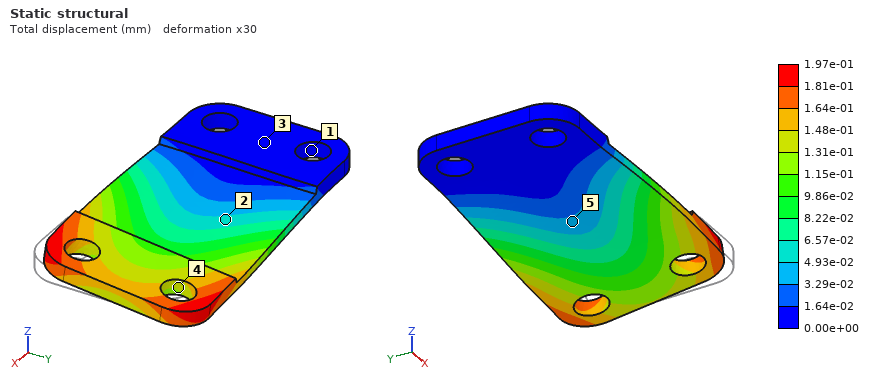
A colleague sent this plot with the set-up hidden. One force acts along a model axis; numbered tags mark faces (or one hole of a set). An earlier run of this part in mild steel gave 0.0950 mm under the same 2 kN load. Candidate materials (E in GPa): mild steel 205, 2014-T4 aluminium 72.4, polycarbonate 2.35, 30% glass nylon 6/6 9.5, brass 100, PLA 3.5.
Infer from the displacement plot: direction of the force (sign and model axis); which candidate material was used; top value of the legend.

+Y
brass
1.97e-01 mm
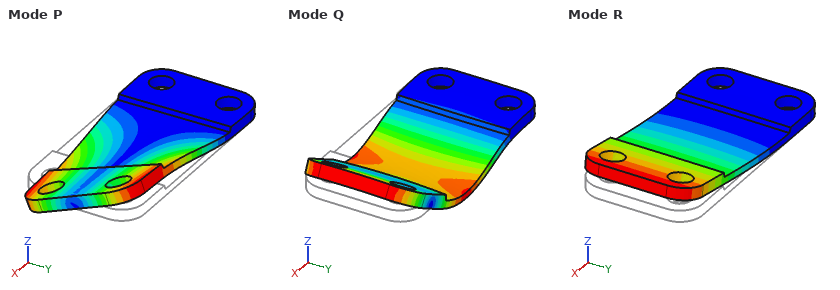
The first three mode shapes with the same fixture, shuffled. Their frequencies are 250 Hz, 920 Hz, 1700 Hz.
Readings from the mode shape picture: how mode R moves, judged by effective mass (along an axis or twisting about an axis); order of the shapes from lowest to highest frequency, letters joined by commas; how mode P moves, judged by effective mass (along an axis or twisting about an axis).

along Z
R, P, Q
twisting about X
